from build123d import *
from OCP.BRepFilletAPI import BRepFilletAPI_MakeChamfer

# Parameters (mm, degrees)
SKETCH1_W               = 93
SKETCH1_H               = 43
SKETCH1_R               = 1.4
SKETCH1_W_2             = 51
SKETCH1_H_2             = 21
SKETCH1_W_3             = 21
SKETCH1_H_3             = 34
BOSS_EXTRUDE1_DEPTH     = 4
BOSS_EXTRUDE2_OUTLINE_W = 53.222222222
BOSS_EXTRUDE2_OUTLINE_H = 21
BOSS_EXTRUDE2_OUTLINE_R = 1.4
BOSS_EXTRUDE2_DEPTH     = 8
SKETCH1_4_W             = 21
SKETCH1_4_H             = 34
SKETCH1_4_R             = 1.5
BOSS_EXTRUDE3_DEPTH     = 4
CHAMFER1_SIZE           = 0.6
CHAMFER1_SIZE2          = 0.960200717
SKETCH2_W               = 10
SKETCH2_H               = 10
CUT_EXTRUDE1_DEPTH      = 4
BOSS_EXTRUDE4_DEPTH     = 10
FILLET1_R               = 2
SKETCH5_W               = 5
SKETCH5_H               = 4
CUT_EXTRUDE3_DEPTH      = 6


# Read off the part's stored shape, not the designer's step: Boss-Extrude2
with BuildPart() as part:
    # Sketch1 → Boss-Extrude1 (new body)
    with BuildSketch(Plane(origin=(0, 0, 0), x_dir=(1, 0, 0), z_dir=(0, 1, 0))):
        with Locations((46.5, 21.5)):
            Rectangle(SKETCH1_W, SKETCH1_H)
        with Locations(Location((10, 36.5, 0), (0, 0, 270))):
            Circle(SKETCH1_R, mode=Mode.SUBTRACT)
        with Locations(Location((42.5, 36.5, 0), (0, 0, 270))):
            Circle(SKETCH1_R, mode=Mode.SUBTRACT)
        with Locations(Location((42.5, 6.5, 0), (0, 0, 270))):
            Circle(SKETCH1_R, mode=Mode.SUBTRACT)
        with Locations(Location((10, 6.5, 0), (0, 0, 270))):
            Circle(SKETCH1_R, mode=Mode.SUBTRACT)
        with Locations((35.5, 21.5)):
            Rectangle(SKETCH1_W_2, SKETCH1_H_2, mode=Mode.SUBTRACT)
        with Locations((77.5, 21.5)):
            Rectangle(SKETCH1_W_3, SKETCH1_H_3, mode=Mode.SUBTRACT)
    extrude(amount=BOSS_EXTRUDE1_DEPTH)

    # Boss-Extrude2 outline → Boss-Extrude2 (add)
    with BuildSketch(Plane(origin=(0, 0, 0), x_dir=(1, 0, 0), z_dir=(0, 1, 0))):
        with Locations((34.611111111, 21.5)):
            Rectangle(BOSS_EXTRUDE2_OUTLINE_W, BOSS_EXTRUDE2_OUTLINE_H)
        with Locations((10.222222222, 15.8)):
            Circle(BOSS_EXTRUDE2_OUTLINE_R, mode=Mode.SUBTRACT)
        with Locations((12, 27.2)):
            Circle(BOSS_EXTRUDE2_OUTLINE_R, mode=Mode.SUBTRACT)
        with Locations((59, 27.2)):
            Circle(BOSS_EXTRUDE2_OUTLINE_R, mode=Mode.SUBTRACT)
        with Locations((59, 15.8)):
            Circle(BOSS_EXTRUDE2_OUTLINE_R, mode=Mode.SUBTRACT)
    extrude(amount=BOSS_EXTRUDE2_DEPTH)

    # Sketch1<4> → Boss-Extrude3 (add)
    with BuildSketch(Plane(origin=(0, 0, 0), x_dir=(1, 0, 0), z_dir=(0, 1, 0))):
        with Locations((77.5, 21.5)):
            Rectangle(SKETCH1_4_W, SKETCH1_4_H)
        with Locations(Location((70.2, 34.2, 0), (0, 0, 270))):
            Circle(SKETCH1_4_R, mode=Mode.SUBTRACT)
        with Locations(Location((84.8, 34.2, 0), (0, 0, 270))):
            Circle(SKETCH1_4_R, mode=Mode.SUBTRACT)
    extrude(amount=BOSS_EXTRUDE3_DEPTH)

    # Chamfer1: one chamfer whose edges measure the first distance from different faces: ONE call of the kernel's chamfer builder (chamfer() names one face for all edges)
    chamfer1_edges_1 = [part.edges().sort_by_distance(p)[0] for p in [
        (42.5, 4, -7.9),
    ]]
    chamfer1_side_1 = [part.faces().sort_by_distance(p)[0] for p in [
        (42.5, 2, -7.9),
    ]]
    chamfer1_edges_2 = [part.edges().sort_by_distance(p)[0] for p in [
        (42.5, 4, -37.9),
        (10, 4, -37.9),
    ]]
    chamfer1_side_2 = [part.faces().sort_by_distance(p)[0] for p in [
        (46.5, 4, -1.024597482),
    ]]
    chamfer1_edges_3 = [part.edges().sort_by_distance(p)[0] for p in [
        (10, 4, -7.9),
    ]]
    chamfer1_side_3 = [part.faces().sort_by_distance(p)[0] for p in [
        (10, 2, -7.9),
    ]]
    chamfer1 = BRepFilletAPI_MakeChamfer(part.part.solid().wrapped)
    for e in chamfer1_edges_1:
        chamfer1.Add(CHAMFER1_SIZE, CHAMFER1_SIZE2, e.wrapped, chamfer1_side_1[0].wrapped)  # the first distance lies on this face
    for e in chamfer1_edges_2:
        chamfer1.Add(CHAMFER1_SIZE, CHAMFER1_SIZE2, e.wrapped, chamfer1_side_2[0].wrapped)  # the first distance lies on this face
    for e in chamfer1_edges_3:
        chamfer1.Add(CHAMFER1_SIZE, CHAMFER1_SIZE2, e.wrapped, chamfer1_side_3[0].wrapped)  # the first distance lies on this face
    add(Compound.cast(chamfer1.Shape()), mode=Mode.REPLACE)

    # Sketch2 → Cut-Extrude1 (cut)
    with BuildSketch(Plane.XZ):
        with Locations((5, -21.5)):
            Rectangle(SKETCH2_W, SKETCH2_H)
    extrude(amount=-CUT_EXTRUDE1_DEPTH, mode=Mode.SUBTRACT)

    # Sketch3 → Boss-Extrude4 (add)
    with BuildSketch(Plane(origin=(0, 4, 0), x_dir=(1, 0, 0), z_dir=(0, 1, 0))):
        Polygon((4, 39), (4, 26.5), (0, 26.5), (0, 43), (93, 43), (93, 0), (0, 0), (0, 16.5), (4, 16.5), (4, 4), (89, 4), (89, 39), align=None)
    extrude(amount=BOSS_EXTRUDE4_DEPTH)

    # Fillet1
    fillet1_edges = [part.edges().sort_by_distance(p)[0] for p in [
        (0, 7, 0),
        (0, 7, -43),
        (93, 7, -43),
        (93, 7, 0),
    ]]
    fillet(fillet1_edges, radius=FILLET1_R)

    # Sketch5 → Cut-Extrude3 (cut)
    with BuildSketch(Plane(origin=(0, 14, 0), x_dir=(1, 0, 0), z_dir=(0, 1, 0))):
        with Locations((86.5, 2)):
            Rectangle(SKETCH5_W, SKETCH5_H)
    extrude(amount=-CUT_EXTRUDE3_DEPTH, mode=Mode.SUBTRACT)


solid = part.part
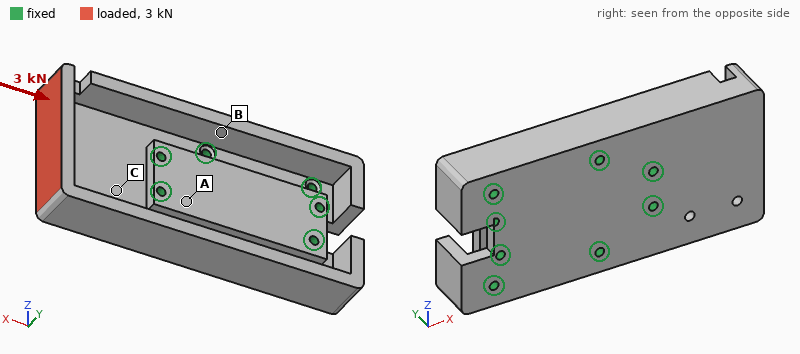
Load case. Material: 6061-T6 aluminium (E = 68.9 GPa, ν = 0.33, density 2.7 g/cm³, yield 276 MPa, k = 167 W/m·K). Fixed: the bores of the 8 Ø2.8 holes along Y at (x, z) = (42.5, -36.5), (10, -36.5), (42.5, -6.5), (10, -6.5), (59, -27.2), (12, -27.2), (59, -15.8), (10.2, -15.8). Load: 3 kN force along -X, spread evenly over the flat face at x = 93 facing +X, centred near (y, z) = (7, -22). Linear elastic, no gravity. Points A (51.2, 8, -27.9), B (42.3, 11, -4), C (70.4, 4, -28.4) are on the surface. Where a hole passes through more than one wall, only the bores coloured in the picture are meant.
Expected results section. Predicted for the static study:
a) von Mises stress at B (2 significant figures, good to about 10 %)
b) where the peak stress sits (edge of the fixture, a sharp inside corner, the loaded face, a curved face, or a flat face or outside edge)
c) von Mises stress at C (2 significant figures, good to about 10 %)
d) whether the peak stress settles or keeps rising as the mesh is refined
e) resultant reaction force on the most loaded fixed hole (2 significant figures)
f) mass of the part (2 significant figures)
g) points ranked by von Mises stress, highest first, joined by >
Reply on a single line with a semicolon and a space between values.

14 MPa; a sharp inside corner; 26 MPa; keeps rising; 770 N; 79 g; C > B > A
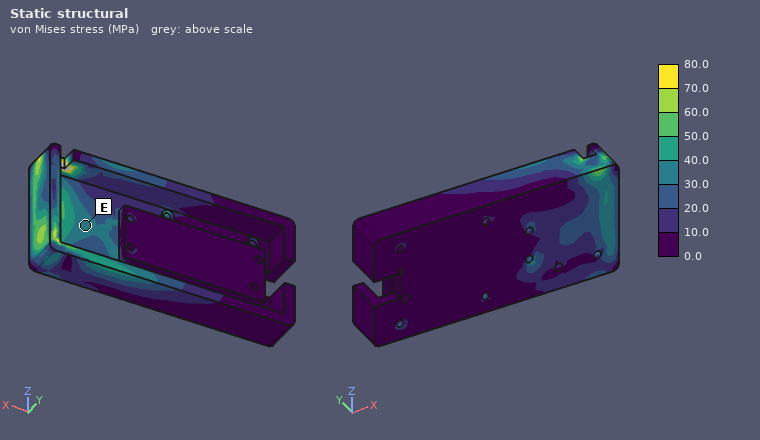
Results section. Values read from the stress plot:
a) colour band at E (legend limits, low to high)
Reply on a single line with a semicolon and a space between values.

30.0 to 40.0 MPa
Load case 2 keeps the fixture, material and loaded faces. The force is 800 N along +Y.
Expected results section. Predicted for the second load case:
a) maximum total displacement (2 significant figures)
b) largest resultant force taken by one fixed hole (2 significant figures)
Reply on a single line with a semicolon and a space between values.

0.16 mm; 810 N
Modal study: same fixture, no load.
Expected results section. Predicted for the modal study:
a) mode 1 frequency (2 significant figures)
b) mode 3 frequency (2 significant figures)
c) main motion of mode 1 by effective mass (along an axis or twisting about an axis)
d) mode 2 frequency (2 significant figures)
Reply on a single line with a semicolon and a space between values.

3700 Hz; 10 kHz; along Y; 4400 Hz
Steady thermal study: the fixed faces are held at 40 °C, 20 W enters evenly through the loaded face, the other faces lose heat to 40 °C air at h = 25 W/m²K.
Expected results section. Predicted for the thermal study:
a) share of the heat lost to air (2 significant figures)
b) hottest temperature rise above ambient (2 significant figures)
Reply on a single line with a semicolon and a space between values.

7.3 %; 21 K
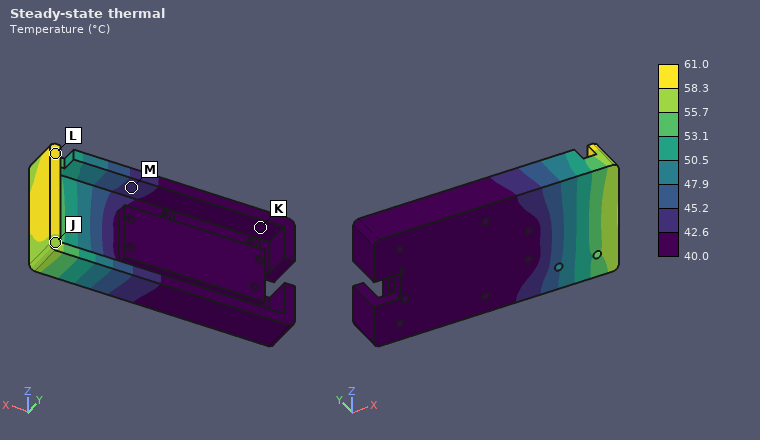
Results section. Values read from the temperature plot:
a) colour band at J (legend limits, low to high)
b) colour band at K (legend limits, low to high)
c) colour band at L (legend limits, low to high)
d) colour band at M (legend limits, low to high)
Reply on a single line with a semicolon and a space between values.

55.7 to 58.3 °C; 40.0 to 42.6 °C; 58.3 to 61.0 °C; 42.6 to 45.2 °C
